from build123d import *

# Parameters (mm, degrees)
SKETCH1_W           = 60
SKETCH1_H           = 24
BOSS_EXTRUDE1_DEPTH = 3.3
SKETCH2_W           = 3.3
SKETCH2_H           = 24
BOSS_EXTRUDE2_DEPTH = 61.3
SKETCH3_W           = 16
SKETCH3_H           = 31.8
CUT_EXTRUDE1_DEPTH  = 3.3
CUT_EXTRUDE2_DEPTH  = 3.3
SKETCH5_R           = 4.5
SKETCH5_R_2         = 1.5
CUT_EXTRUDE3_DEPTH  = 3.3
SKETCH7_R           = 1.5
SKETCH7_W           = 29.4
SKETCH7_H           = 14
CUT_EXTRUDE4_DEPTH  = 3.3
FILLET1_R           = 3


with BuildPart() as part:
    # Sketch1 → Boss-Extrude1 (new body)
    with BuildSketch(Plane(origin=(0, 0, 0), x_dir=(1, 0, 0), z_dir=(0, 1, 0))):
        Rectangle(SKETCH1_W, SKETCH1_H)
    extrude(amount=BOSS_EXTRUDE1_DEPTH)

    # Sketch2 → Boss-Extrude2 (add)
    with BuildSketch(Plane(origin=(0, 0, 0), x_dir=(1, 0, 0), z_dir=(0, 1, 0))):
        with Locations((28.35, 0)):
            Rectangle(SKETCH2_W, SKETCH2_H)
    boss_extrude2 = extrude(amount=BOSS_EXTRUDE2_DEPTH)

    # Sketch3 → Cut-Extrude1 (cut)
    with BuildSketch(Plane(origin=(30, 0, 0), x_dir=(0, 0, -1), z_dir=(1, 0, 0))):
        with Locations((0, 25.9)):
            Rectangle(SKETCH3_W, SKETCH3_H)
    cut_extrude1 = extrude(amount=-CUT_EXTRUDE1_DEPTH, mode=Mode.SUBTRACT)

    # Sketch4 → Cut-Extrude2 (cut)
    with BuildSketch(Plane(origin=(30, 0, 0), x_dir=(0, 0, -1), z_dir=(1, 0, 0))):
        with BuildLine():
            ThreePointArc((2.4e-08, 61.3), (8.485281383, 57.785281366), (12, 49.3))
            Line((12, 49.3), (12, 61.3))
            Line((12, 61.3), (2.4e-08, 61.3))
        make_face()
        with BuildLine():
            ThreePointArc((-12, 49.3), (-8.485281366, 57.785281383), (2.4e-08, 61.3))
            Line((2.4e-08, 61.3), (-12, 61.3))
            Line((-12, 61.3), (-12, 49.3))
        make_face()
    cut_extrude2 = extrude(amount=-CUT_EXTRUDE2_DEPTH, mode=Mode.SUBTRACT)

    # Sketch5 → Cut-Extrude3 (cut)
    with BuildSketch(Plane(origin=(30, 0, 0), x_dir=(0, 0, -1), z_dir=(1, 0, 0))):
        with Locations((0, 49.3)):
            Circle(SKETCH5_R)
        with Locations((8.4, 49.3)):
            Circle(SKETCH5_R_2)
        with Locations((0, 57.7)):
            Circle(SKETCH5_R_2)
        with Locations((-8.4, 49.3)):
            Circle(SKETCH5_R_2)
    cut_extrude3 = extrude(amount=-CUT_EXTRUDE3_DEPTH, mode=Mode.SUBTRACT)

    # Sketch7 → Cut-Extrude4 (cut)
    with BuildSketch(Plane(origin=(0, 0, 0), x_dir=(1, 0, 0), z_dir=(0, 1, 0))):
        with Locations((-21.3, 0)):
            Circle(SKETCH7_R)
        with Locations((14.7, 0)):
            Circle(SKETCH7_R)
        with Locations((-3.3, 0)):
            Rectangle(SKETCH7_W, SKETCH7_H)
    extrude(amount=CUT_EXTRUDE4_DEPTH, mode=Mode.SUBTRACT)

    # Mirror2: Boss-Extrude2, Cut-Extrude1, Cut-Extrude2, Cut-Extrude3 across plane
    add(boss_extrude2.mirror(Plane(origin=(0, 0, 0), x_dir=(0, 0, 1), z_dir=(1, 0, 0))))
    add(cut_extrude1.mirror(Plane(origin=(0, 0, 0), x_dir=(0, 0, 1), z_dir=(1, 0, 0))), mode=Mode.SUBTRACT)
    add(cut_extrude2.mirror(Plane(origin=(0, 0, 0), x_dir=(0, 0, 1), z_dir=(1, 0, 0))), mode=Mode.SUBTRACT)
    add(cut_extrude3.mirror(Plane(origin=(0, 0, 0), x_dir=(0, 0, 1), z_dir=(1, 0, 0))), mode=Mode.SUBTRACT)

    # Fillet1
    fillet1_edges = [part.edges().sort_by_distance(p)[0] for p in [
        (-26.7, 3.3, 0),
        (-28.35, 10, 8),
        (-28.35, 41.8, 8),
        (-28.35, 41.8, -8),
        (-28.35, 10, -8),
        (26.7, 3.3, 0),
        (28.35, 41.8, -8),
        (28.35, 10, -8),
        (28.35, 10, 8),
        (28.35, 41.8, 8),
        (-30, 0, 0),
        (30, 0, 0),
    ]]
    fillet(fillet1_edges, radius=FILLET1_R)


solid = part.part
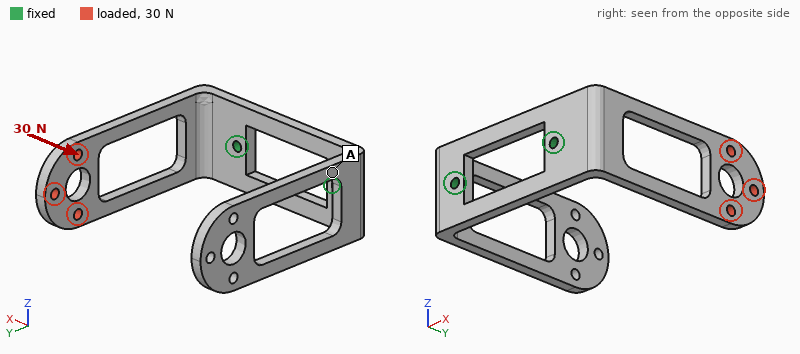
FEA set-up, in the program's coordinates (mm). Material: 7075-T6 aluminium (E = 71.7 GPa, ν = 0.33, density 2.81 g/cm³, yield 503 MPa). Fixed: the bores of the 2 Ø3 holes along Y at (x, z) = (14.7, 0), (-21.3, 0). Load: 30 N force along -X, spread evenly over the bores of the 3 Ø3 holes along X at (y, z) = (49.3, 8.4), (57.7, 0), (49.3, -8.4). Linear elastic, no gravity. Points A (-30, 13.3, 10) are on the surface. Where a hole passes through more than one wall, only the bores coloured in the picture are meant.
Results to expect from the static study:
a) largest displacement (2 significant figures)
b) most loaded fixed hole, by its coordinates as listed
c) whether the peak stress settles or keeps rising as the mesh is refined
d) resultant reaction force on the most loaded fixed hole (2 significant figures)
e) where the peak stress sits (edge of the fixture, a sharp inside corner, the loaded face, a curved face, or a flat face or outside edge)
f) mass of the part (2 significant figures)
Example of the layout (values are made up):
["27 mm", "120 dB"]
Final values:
["0.94 mm", "(14.7, 0)", "keeps rising", "32 N", "edge of the fixture", "23 g"]
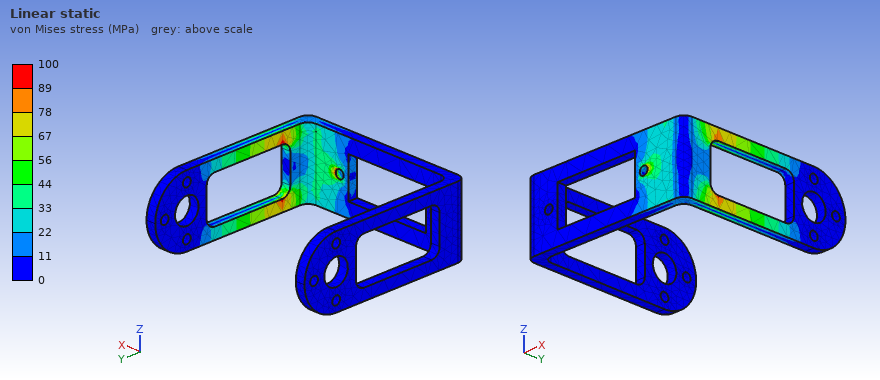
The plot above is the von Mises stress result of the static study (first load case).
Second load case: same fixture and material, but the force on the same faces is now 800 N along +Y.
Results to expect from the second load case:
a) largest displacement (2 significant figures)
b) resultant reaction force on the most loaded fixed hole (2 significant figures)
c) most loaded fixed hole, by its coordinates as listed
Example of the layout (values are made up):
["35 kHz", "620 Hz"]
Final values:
["1.0 mm", "860 N", "(14.7, 0)"]
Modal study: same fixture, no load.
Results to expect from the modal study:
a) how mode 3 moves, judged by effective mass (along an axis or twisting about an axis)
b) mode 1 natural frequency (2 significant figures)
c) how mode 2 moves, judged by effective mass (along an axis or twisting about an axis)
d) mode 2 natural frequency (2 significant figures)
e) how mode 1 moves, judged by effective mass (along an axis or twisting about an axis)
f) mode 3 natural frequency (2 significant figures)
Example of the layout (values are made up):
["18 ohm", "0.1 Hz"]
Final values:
["along Z", "570 Hz", "along X", "610 Hz", "along X", "1100 Hz"]
